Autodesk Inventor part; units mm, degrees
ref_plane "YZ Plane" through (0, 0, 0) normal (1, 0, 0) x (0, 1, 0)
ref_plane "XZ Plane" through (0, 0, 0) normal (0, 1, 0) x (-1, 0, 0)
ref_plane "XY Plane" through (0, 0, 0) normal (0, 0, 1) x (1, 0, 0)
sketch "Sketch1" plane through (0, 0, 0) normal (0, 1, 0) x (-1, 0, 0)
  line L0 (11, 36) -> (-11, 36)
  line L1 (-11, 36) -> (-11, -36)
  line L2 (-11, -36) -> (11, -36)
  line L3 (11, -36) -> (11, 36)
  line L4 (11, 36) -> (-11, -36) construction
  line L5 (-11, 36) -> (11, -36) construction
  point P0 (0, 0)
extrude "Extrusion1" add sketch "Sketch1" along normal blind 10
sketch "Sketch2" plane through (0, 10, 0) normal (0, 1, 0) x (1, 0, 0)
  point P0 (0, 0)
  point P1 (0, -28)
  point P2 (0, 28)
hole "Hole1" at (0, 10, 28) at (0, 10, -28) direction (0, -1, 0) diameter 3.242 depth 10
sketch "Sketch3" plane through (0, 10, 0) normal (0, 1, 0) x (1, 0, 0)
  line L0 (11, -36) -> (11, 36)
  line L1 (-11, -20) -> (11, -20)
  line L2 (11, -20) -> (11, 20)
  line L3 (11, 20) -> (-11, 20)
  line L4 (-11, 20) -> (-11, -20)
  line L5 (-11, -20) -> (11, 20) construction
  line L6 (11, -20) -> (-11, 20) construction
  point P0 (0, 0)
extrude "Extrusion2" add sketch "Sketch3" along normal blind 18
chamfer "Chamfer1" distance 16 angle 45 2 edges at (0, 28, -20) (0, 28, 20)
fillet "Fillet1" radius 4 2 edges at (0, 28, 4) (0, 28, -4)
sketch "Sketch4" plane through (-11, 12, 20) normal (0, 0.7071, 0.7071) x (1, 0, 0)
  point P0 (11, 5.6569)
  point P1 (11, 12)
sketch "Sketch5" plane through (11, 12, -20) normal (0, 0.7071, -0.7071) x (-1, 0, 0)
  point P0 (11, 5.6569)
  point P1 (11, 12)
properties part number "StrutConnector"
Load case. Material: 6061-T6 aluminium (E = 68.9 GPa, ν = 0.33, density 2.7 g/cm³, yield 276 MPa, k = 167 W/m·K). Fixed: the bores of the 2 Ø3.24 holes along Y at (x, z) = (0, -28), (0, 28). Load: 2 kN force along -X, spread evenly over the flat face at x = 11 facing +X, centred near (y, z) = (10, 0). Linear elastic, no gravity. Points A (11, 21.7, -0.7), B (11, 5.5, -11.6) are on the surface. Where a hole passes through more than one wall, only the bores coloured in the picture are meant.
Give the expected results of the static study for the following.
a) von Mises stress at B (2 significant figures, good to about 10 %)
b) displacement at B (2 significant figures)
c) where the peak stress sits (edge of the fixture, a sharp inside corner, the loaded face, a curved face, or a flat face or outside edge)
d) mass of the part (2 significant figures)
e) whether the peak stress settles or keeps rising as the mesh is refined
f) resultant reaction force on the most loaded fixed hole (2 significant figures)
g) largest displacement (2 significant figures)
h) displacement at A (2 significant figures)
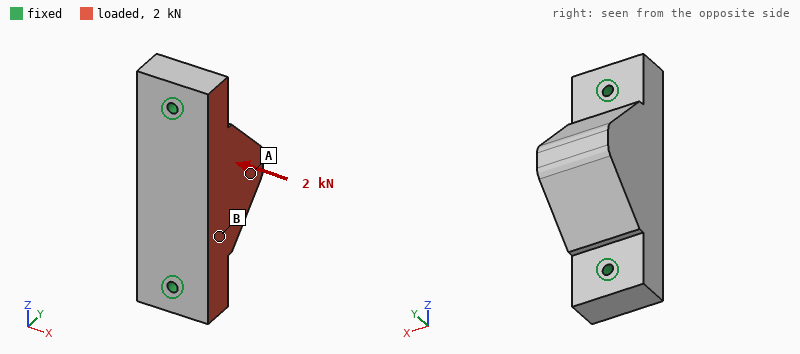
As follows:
8.7 MPa
7.7 µm
edge of the fixture
70 g
keeps rising
1.0 kN
19 µm
16 µm
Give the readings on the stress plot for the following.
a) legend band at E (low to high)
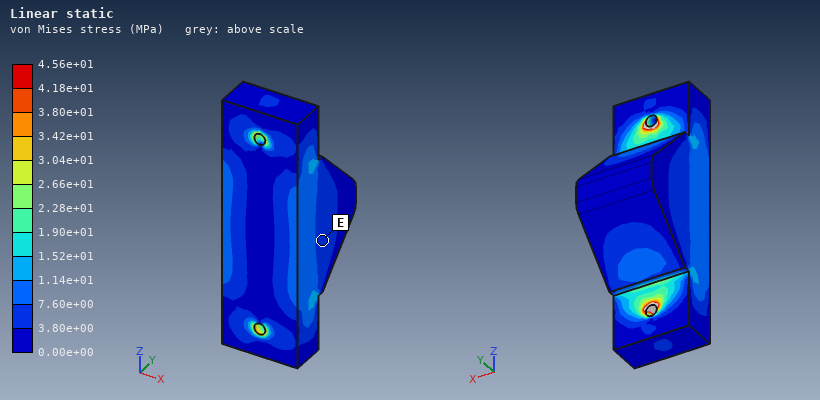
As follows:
3.80e+00 to 7.60e+00 MPa
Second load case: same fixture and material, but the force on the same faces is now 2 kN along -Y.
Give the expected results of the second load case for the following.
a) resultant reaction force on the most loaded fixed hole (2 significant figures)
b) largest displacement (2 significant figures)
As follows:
1.1 kN
29 µm
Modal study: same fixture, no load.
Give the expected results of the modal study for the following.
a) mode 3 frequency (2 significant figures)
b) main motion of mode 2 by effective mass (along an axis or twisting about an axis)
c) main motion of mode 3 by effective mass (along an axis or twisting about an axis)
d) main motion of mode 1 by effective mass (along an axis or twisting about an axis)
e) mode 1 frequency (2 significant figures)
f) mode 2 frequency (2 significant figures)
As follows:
15 kHz
along Y
along X
along X
7400 Hz
12 kHz
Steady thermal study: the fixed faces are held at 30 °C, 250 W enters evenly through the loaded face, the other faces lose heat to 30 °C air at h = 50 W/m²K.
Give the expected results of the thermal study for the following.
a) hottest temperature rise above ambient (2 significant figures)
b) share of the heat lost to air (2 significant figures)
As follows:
63 K
3.4 %
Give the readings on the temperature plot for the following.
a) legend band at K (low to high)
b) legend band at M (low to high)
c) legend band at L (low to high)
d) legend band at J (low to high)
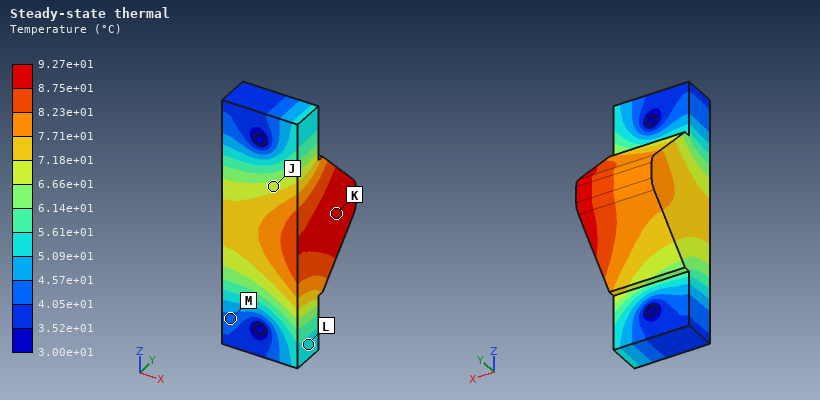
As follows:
8.75e+01 to 9.27e+01 °C
4.05e+01 to 4.57e+01 °C
5.09e+01 to 5.61e+01 °C
6.66e+01 to 7.18e+01 °C
